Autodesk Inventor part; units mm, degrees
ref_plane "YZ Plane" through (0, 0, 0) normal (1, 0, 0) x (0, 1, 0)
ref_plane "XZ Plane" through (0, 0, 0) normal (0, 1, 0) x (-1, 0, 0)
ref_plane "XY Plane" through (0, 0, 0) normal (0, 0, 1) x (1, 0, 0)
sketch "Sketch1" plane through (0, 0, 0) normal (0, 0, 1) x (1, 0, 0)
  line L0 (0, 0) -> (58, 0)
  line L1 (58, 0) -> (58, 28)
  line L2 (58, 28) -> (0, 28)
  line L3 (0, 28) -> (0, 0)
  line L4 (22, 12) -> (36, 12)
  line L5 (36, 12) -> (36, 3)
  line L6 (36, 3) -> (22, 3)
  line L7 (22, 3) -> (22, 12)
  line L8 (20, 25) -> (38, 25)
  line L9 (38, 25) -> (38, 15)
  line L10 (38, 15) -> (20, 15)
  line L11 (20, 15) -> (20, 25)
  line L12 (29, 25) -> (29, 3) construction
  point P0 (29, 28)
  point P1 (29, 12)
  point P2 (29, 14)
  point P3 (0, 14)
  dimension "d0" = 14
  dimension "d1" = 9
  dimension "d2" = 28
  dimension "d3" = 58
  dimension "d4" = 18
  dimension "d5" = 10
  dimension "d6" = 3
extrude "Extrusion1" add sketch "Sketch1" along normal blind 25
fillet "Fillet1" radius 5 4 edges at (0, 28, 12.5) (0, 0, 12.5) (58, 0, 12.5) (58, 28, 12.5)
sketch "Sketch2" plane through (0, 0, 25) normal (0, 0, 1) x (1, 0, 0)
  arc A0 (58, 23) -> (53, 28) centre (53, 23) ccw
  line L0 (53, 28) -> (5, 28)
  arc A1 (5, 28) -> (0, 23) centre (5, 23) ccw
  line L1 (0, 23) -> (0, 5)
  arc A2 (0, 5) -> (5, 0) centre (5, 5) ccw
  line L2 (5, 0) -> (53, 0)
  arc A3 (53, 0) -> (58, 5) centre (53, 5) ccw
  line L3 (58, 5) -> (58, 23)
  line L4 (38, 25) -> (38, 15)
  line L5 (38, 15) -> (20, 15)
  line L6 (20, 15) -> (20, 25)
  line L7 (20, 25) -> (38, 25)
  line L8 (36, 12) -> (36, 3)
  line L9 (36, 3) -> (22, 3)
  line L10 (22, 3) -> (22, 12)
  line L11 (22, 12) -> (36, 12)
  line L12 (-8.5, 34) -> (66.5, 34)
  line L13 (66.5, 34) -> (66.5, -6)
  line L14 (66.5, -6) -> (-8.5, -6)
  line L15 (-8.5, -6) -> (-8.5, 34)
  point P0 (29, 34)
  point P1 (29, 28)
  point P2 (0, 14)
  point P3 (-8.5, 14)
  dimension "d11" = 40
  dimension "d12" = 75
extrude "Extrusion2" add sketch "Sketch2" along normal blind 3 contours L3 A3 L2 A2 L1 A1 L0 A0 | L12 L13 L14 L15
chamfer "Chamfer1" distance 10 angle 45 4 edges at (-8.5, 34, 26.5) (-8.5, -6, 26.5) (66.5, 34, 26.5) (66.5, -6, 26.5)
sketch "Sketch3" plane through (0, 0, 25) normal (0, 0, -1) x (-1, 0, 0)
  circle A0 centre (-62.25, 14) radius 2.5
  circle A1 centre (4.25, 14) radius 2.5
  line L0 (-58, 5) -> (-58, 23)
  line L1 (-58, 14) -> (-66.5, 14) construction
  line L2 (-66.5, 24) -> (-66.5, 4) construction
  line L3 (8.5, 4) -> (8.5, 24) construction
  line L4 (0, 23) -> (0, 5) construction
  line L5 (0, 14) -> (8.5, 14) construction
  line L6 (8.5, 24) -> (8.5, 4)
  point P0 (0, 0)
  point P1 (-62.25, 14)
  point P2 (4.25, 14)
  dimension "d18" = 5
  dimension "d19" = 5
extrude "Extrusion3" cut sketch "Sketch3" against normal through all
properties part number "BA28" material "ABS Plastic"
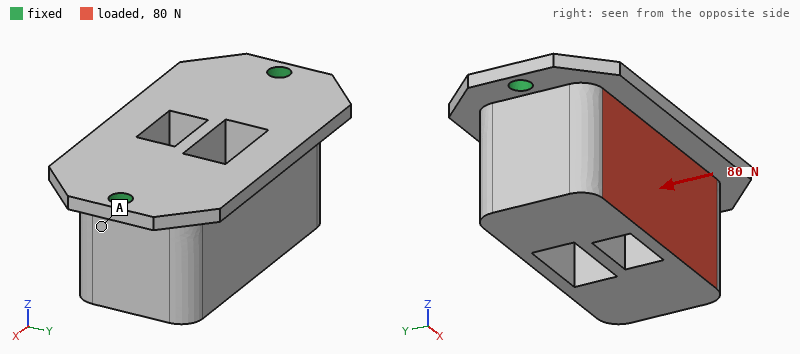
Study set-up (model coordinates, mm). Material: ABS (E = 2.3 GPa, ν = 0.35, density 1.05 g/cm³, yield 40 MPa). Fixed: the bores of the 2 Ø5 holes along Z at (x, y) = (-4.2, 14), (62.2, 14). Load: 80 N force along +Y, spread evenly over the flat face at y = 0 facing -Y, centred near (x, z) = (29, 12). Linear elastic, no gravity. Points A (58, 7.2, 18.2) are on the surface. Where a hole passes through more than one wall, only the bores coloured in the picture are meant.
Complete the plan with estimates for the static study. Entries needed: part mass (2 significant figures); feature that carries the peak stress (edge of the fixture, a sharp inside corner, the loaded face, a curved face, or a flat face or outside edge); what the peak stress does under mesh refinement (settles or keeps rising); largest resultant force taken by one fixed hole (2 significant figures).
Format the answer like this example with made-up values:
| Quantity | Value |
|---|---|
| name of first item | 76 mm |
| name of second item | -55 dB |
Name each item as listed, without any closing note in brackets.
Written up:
| Quantity | Value |
|---|---|
| part mass | 42 g |
| feature that carries the peak stress | edge of the fixture |
| what the peak stress does under mesh refinement | keeps rising |
| largest resultant force taken by one fixed hole | 40 N |
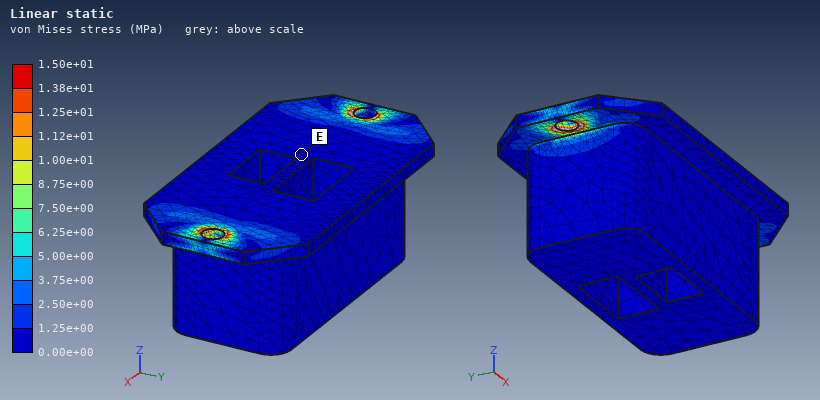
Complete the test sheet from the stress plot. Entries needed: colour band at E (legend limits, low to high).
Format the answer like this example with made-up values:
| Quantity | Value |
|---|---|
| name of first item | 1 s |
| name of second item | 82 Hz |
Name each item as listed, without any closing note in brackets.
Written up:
| Quantity | Value |
|---|---|
| colour band at E | 0.00e+00 to 1.25e+00 MPa |
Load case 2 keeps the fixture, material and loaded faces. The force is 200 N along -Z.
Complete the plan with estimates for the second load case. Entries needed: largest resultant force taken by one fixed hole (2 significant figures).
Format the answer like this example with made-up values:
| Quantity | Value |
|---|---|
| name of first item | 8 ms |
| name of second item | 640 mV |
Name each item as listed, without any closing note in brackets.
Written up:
| Quantity | Value |
|---|---|
| largest resultant force taken by one fixed hole | 120 N |
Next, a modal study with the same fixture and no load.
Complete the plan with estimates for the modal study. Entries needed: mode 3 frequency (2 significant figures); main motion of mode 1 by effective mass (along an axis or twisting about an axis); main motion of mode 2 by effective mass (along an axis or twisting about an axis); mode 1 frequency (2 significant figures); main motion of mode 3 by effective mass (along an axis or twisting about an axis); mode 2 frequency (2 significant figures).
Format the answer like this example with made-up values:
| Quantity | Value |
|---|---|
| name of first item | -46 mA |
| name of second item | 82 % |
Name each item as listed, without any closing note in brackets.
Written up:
| Quantity | Value |
|---|---|
| mode 3 frequency | 2600 Hz |
| main motion of mode 1 by effective mass | along Y |
| main motion of mode 2 by effective mass | along Z |
| mode 1 frequency | 480 Hz |
| main motion of mode 3 by effective mass | along X |
| mode 2 frequency | 2000 Hz |
